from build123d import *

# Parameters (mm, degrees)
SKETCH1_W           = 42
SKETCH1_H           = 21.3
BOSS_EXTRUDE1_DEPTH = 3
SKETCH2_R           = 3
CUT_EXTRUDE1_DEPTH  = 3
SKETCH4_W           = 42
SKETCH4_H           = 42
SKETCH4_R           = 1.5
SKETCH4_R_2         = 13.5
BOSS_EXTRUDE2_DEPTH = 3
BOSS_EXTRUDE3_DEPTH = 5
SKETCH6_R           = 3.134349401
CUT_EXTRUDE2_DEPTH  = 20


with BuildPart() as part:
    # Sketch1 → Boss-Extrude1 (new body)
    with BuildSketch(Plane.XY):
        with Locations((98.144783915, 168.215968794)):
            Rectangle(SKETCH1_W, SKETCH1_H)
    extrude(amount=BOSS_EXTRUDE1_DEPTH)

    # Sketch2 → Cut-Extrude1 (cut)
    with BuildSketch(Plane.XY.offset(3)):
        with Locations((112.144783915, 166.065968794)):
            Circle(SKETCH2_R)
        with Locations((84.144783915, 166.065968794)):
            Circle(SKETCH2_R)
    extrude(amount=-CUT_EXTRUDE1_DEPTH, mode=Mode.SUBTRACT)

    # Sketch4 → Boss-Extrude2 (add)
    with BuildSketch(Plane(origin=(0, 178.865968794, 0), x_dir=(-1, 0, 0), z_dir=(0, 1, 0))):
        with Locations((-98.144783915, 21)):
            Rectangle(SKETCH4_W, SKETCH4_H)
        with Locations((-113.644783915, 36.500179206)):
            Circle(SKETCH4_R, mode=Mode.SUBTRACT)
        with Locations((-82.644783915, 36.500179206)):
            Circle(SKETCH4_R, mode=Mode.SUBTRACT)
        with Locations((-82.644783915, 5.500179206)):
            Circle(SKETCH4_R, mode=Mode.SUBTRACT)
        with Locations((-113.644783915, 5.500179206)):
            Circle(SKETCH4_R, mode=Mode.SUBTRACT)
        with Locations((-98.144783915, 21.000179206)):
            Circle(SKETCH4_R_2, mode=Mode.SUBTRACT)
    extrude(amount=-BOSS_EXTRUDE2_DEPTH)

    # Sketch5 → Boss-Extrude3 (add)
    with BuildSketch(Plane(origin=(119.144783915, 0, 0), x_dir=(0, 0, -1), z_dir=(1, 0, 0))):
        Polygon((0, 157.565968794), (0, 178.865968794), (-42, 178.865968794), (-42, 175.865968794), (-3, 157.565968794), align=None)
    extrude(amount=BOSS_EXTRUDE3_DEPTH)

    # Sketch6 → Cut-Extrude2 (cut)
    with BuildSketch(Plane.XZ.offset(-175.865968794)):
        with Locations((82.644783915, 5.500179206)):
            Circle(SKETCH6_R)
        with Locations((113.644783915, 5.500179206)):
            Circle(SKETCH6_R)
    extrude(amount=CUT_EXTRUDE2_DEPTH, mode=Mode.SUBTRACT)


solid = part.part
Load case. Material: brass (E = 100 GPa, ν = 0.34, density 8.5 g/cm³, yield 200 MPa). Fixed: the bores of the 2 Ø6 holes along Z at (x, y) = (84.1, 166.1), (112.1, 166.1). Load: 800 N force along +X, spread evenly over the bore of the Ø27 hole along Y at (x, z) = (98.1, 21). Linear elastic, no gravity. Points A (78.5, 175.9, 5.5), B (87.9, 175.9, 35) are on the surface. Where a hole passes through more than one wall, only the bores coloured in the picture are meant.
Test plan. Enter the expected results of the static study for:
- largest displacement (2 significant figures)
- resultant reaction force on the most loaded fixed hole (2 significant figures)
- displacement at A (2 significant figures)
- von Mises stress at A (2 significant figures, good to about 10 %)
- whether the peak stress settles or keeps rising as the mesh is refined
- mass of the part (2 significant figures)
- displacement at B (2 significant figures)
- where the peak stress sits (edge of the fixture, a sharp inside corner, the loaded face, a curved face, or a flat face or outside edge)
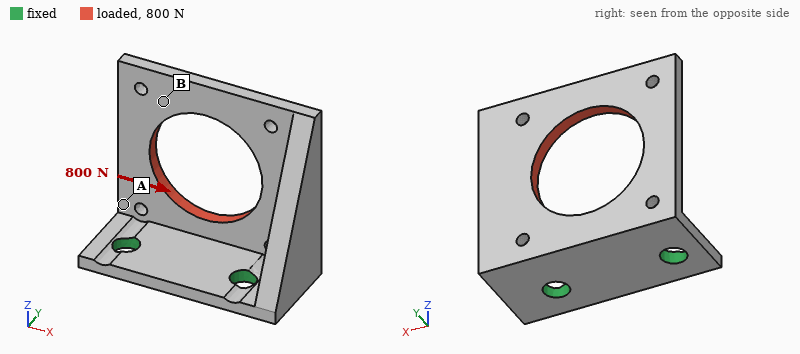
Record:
0.13 mm
670 N
0.037 mm
70 MPa
keeps rising
70 g
0.086 mm
edge of the fixture
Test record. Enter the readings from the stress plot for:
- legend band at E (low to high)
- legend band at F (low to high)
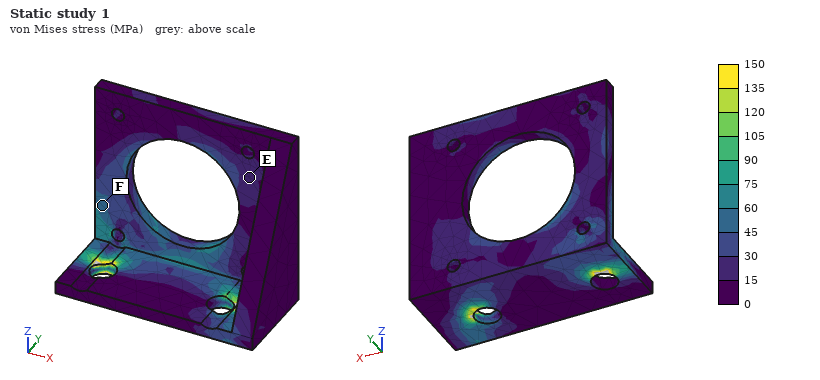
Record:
15 to 30 MPa
45 to 60 MPa
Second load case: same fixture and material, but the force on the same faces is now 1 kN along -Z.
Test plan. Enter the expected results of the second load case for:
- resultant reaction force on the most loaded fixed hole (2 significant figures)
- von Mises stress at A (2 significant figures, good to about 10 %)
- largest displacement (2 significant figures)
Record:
510 N
35 MPa
0.16 mm
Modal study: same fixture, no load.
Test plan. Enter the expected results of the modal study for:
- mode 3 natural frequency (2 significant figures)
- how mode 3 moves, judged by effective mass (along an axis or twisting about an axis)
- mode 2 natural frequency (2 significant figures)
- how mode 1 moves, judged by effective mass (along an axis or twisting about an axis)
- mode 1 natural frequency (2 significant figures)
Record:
3100 Hz
along X
1800 Hz
along Y
1100 Hz
